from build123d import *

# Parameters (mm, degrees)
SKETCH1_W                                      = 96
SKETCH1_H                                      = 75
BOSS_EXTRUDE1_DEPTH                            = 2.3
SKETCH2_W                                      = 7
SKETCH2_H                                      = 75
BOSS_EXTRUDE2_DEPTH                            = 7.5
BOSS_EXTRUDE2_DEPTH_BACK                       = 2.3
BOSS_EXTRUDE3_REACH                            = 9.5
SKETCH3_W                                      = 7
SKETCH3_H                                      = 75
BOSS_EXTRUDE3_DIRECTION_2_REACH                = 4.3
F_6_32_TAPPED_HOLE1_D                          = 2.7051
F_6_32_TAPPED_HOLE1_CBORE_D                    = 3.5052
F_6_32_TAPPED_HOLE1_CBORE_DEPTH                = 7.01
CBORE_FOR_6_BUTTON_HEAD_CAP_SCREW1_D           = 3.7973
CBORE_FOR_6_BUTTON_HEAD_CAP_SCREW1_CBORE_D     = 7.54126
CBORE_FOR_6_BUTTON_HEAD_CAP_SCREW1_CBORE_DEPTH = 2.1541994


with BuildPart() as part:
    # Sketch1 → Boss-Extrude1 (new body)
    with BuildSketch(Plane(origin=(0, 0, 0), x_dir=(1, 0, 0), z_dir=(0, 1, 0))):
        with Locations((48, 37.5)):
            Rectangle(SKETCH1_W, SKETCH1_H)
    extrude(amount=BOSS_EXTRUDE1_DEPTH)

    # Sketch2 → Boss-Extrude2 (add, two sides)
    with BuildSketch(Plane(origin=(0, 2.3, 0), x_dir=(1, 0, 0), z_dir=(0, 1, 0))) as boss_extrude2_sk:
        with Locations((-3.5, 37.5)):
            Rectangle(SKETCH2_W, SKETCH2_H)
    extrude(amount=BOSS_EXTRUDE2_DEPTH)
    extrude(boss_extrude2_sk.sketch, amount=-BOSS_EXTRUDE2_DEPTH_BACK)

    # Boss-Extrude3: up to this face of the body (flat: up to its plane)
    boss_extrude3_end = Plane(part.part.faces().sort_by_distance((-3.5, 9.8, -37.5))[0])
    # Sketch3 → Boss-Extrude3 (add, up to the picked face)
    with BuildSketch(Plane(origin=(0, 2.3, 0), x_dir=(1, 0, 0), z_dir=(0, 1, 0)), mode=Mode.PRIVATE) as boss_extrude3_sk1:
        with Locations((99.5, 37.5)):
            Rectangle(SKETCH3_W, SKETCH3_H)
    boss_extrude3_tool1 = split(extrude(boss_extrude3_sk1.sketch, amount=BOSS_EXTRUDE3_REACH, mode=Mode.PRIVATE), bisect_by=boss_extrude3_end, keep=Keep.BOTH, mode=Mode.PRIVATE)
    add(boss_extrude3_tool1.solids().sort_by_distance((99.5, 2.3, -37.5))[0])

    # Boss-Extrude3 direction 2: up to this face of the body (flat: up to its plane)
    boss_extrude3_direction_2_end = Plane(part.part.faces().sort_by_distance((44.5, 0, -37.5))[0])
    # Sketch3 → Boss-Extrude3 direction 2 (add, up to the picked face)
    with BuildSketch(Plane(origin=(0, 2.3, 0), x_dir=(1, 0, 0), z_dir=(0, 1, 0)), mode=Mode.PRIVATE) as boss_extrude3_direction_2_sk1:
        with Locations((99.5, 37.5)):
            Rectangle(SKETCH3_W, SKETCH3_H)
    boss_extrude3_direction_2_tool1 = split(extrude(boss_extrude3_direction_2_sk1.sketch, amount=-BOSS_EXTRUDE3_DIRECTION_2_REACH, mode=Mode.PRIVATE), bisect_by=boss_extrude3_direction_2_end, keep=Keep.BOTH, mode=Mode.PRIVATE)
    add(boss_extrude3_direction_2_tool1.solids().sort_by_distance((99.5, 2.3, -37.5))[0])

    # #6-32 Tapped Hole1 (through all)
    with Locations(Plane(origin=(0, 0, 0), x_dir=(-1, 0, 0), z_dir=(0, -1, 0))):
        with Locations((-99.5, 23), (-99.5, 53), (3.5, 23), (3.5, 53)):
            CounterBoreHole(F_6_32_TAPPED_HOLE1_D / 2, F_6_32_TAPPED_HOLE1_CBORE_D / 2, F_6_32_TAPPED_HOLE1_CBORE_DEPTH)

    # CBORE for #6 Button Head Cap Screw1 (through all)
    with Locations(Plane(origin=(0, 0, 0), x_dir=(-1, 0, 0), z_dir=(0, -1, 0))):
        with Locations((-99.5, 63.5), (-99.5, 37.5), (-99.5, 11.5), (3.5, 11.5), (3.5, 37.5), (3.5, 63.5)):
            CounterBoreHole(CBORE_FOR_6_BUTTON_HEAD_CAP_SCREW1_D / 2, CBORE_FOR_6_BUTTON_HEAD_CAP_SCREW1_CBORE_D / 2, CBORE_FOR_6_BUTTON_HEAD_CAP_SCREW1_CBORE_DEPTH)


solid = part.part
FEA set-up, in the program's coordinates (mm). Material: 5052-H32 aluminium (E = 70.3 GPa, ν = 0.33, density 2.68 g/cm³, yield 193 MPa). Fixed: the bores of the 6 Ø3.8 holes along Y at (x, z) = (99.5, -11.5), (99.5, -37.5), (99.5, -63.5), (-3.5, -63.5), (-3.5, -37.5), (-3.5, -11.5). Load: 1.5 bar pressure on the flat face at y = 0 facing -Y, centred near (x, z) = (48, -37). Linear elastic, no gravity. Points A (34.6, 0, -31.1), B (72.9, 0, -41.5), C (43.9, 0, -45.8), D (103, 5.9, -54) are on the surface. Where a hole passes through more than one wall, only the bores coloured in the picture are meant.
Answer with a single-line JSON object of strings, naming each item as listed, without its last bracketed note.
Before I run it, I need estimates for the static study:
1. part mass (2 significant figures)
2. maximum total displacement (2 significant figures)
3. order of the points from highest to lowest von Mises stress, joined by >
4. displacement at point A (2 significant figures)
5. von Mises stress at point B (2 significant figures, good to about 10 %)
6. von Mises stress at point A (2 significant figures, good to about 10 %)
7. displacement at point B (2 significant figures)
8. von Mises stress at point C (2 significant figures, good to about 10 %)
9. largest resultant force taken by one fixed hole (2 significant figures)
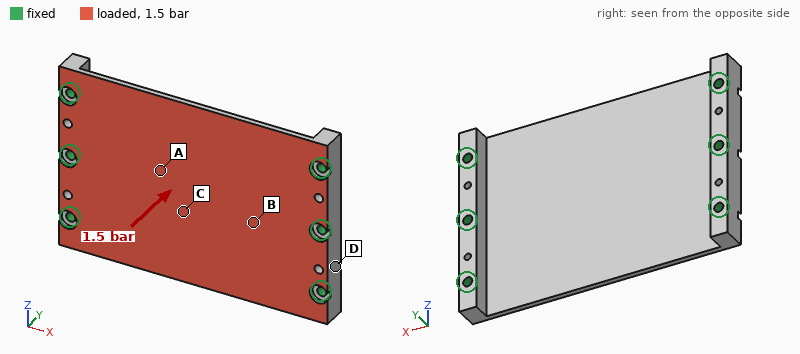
{"part mass": "68 g", "maximum total displacement": "0.56 mm", "order of the points from highest to lowest von Mises stress, joined by >": "C > A > B > D", "displacement at point A": "0.43 mm", "von Mises stress at point B": "22 MPa", "von Mises stress at point A": "54 MPa", "displacement at point B": "0.28 mm", "von Mises stress at point C": "66 MPa", "largest resultant force taken by one fixed hole": "360 N"}
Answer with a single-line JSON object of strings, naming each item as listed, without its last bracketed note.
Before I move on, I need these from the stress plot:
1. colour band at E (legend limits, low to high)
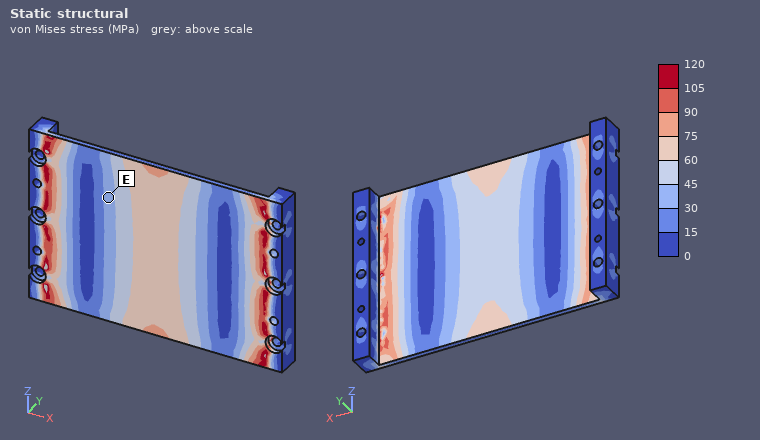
{"colour band at E": "30 to 45 MPa"}
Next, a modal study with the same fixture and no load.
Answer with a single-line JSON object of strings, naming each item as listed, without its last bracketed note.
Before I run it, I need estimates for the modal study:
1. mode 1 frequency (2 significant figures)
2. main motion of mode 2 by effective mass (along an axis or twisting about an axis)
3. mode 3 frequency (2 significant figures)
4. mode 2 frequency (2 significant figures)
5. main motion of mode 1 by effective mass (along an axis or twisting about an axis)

{"mode 1 frequency": "1200 Hz", "main motion of mode 2 by effective mass": "twisting about X", "mode 3 frequency": "3400 Hz", "mode 2 frequency": "1600 Hz", "main motion of mode 1 by effective mass": "along Y"}
